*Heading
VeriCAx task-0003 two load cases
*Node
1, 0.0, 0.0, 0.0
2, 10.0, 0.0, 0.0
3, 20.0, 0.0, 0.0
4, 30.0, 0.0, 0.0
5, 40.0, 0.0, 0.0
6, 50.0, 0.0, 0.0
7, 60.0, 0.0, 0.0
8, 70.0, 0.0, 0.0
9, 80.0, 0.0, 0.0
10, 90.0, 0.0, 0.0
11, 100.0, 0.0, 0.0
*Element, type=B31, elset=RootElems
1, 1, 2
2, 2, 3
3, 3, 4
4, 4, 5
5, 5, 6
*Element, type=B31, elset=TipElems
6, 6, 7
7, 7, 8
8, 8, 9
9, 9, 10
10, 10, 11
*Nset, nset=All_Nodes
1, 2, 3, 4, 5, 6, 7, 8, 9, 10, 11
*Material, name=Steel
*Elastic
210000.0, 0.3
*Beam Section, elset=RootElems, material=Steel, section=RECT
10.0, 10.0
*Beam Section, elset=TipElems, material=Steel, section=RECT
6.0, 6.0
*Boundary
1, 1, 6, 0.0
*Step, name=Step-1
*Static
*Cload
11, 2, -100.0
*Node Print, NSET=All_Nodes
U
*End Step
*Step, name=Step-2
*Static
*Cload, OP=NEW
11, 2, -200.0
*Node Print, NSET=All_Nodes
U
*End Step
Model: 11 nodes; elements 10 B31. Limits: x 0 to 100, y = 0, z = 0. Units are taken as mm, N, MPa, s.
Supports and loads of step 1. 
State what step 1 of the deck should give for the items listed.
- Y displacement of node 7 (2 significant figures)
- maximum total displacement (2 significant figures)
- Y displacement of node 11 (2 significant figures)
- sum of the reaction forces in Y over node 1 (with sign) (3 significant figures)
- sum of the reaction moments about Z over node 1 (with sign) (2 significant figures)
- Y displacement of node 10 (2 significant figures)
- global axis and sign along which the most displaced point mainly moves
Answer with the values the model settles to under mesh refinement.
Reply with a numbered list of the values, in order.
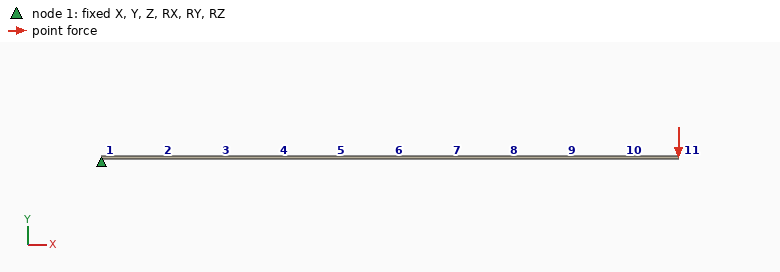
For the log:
1. -0.092 mm
2. 0.35 mm
3. -0.35 mm
4. 100 N
5. 10000 N·mm
6. -0.28 mm
7. -Y
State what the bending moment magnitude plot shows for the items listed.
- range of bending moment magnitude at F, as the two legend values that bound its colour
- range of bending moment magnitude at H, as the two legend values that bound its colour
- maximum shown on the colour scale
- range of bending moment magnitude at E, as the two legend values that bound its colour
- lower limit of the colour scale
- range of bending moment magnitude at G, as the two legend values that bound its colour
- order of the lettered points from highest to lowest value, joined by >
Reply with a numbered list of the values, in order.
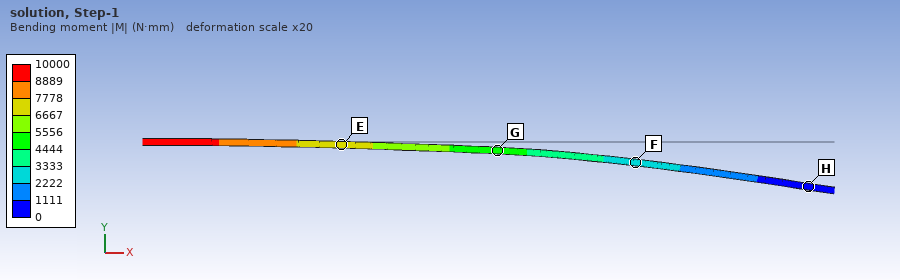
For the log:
1. 2222 to 3333 N·mm
2. 0 to 1111 N·mm
3. 10000 N·mm
4. 6667 to 7778 N·mm
5. 0 N·mm
6. 4444 to 5556 N·mm
7. E > G > F > H
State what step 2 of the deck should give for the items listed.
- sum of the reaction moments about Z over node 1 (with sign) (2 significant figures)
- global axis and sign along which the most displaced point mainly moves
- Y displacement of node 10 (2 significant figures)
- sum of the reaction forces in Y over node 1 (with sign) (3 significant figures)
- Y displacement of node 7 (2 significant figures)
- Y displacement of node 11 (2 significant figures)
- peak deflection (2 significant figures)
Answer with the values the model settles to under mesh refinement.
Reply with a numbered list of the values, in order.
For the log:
1. 20000 N·mm
2. -Y
3. -0.55 mm
4. 200 N
5. -0.18 mm
6. -0.71 mm
7. 0.71 mm
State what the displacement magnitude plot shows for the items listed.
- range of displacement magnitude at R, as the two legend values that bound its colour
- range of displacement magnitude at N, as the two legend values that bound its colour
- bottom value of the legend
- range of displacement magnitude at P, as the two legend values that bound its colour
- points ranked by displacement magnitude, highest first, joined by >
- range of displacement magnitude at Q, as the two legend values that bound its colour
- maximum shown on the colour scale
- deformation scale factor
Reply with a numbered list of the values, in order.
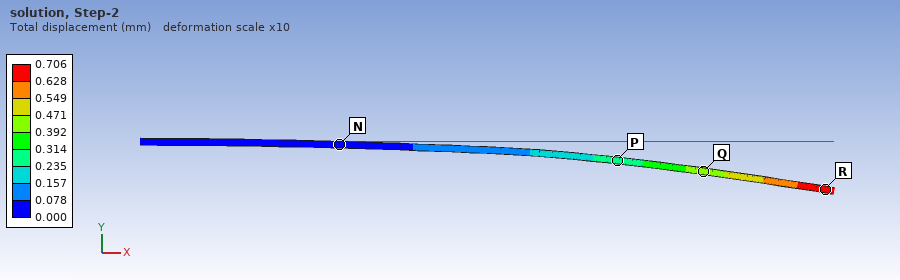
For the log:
1. 0.628 to 0.706 mm
2. 0.000 to 0.078 mm
3. 0.000 mm
4. 0.235 to 0.314 mm
5. R > Q > P > N
6. 0.392 to 0.471 mm
7. 0.706 mm
8. 10
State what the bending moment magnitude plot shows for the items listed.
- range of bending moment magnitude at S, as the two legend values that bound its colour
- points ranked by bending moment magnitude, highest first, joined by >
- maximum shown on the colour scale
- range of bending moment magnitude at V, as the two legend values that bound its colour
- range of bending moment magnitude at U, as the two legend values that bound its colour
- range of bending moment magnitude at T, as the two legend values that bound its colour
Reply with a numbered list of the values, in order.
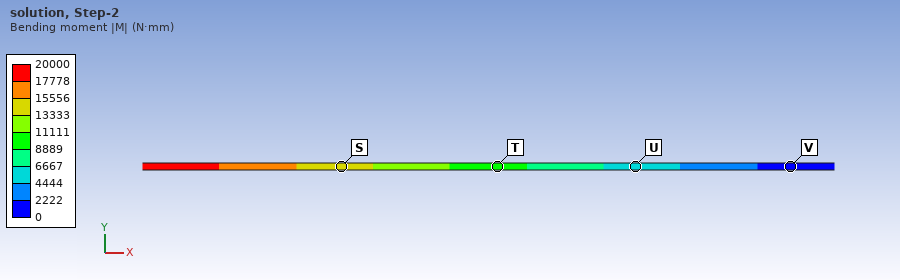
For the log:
1. 13333 to 15556 N·mm
2. S > T > U > V
3. 20000 N·mm
4. 0 to 2222 N·mm
5. 4444 to 6667 N·mm
6. 8889 to 11111 N·mm
